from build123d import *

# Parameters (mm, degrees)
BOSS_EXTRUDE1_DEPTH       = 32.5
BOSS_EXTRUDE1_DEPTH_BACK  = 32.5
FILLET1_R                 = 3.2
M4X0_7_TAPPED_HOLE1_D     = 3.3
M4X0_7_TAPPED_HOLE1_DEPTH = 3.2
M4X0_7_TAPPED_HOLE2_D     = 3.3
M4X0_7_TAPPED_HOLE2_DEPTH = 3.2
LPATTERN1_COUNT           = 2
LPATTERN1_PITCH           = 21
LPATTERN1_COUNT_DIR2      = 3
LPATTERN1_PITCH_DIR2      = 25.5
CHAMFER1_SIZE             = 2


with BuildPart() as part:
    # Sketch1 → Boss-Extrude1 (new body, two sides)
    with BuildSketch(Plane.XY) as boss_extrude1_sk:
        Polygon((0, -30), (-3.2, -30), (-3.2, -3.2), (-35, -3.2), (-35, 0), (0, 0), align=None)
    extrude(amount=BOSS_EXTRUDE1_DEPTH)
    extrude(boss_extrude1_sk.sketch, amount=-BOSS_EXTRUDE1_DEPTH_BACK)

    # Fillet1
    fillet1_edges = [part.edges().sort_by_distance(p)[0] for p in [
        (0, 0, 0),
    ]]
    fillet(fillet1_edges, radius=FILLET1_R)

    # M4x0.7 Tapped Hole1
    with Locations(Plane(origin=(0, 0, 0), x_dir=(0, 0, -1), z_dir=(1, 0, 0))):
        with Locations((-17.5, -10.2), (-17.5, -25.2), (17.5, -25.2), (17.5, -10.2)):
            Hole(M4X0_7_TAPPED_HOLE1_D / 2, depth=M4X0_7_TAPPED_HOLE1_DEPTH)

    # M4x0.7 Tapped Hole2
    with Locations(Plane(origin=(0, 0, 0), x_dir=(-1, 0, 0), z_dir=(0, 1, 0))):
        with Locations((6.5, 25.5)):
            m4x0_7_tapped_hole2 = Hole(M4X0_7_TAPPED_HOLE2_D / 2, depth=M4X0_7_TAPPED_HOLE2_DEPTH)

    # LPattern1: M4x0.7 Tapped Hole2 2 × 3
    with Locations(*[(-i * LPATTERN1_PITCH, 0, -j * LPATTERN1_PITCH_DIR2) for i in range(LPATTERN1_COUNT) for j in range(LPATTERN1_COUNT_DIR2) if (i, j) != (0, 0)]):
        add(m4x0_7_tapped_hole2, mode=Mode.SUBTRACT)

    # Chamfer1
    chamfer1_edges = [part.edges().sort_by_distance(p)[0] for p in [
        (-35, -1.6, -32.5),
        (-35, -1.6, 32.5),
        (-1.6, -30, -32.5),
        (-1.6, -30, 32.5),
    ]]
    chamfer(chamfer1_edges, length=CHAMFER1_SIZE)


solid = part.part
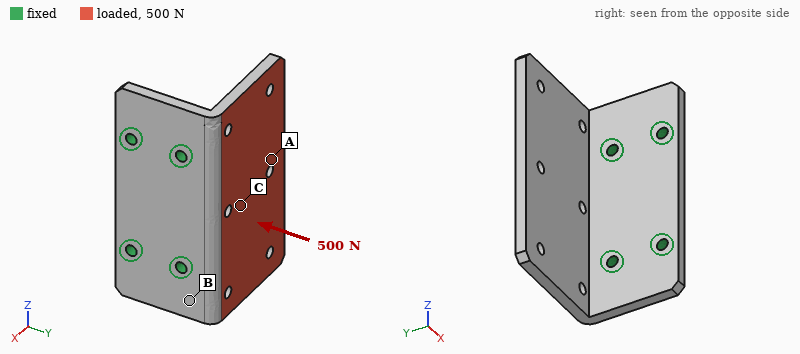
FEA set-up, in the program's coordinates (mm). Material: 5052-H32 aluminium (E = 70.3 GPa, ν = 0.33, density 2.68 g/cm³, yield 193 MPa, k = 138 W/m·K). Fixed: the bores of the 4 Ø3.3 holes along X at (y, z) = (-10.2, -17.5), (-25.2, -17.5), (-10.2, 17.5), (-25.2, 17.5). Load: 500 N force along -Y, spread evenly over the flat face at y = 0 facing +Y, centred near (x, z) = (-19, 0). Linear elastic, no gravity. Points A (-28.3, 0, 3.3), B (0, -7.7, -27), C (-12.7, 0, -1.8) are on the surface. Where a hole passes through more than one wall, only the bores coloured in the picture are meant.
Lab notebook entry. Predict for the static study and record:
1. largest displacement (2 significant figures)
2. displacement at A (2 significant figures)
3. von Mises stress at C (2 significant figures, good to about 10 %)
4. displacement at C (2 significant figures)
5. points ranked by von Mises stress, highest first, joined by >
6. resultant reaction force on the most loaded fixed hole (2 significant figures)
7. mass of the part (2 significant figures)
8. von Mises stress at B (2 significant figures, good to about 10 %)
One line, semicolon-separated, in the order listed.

0.40 mm; 0.31 mm; 29 MPa; 0.11 mm; B > C > A; 230 N; 33 g; 54 MPa
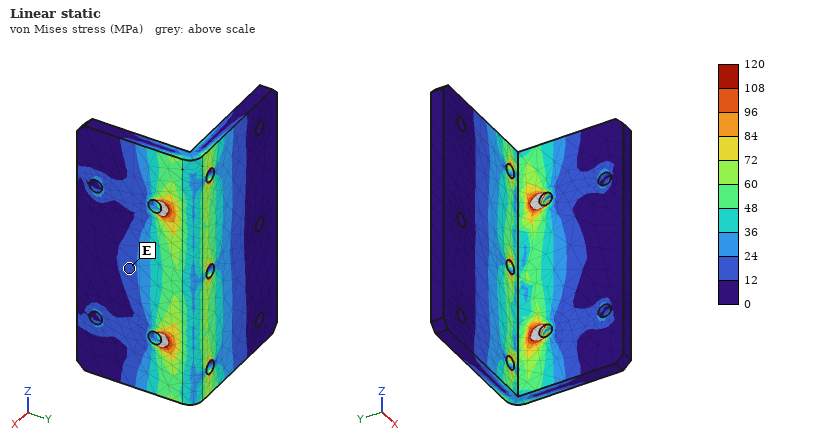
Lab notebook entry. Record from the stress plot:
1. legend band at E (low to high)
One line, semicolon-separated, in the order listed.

12 to 24 MPa
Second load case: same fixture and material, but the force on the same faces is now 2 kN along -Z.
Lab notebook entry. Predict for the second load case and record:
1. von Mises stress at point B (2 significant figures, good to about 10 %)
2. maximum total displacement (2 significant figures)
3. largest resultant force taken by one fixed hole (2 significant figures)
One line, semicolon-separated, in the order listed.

35 MPa; 0.11 mm; 1.5 kN
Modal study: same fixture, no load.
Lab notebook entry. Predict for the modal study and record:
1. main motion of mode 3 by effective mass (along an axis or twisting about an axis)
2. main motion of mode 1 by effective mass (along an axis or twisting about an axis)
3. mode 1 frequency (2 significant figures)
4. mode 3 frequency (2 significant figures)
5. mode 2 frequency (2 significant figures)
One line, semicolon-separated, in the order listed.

along Z; along Y; 1700 Hz; 5800 Hz; 3000 Hz
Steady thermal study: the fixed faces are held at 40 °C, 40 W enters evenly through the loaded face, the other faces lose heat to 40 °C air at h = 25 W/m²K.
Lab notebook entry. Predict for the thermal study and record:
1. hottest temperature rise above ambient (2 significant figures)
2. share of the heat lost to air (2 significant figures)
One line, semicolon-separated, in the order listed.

40 K; 7.0 %
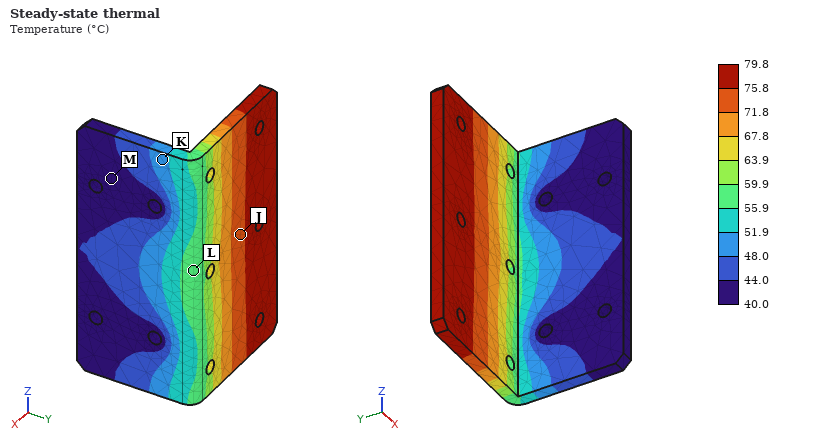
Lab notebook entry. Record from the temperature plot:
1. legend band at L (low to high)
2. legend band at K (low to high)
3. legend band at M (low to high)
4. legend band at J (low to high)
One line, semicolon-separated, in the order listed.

55.9 to 59.9 °C; 48.0 to 51.9 °C; 40.0 to 44.0 °C; 71.8 to 75.8 °C
